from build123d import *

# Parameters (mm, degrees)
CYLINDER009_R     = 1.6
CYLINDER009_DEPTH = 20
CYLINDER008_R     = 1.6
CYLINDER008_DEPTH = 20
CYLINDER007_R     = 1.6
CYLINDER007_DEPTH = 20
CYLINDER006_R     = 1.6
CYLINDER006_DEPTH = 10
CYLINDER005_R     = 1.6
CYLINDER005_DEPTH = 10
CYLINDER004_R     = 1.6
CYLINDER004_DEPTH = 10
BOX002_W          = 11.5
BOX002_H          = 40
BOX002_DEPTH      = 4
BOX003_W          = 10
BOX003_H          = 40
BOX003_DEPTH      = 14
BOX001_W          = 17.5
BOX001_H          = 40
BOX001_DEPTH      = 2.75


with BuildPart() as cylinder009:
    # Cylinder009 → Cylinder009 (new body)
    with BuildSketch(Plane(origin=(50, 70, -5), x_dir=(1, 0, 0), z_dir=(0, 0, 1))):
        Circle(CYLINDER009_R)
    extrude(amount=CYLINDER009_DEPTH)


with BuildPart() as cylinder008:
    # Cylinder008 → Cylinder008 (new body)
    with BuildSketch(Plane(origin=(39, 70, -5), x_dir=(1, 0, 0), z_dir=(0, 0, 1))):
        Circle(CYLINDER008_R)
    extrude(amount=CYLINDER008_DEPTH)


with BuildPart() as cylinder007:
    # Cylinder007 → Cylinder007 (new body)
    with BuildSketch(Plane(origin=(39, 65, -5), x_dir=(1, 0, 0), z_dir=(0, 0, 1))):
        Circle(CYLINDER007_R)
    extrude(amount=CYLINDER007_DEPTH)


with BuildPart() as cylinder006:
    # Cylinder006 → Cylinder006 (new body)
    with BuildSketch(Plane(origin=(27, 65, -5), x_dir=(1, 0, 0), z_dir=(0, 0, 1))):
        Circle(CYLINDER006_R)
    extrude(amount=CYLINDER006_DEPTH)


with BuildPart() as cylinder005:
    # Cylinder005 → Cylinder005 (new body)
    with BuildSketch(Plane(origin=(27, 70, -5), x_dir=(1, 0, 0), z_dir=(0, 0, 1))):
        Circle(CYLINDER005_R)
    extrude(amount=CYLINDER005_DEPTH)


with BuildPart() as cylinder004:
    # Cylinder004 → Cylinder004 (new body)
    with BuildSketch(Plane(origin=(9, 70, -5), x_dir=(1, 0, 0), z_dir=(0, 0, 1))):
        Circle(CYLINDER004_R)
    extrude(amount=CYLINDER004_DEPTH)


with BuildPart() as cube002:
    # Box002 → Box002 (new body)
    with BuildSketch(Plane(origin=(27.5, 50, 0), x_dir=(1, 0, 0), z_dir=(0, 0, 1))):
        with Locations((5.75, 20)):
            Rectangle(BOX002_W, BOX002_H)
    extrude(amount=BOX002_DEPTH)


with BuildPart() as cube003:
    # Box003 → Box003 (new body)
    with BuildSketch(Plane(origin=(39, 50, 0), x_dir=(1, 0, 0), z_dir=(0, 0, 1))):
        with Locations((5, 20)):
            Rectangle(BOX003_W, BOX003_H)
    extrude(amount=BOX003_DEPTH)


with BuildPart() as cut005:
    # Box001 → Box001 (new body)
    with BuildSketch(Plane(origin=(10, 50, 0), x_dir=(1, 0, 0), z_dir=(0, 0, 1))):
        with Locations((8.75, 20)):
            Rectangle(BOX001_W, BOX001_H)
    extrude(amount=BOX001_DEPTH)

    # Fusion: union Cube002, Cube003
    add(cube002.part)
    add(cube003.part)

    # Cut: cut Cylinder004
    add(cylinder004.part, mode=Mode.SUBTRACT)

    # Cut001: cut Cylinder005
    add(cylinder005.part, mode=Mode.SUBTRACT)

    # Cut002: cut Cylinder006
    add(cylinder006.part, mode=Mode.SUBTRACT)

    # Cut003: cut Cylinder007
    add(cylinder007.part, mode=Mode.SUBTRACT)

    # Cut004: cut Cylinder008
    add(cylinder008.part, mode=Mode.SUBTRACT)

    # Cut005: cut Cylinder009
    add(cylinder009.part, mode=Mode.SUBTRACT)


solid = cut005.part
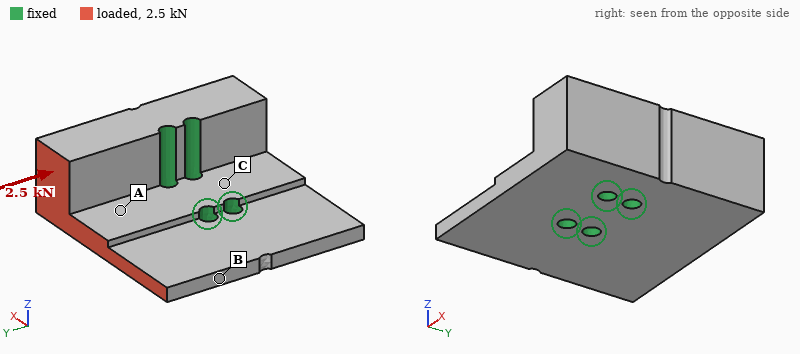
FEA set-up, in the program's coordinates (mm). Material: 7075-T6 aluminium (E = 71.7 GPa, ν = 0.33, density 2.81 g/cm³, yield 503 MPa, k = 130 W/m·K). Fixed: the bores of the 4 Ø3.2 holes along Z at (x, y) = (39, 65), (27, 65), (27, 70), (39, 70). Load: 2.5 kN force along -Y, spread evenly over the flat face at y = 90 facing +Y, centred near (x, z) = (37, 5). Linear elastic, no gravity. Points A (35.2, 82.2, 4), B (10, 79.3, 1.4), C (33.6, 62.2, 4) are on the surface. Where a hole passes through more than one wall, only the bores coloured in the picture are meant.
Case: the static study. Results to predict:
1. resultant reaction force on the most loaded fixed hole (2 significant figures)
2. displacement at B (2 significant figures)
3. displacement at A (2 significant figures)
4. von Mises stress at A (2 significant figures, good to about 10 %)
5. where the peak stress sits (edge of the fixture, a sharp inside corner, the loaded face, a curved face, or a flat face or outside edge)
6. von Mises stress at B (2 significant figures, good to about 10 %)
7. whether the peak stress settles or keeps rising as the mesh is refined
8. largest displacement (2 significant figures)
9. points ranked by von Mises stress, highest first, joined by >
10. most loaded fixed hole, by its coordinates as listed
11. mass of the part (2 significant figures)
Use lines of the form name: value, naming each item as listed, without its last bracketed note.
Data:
resultant reaction force on the most loaded fixed hole: 1.3 kN
displacement at B: 4.4 µm
displacement at A: 2.3 µm
von Mises stress at A: 13 MPa
where the peak stress sits: edge of the fixture
von Mises stress at B: 8.3 MPa
whether the peak stress settles or keeps rising as the mesh is refined: keeps rising
largest displacement: 6.6 µm
points ranked by von Mises stress, highest first, joined by >: A > B > C
most loaded fixed hole, by its coordinates as listed: (39, 70)
mass of the part: 26 g
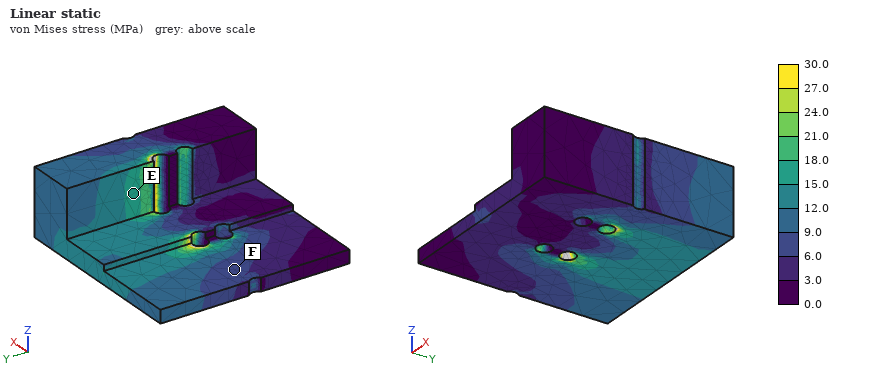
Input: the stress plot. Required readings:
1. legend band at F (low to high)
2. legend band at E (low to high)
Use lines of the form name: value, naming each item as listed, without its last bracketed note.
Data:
legend band at F: 6.0 to 9.0 MPa
legend band at E: 15.0 to 18.0 MPa
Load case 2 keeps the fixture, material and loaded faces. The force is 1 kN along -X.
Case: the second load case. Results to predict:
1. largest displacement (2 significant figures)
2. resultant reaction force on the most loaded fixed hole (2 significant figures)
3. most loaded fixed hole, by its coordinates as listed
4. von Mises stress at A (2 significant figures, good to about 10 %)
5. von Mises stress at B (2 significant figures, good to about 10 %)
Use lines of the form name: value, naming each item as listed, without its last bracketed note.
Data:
largest displacement: 19 µm
resultant reaction force on the most loaded fixed hole: 1.3 kN
most loaded fixed hole, by its coordinates as listed: (39, 70)
von Mises stress at A: 22 MPa
von Mises stress at B: 7.6 MPa
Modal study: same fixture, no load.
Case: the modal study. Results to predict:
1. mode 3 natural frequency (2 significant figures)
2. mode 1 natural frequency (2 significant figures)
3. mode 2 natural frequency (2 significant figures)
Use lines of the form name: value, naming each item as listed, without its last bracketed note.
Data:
mode 3 natural frequency: 14 kHz
mode 1 natural frequency: 6500 Hz
mode 2 natural frequency: 7900 Hz
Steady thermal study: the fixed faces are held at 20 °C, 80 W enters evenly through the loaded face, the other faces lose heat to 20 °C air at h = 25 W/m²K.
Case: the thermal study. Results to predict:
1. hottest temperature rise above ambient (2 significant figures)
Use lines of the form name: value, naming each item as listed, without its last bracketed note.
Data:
hottest temperature rise above ambient: 60 K
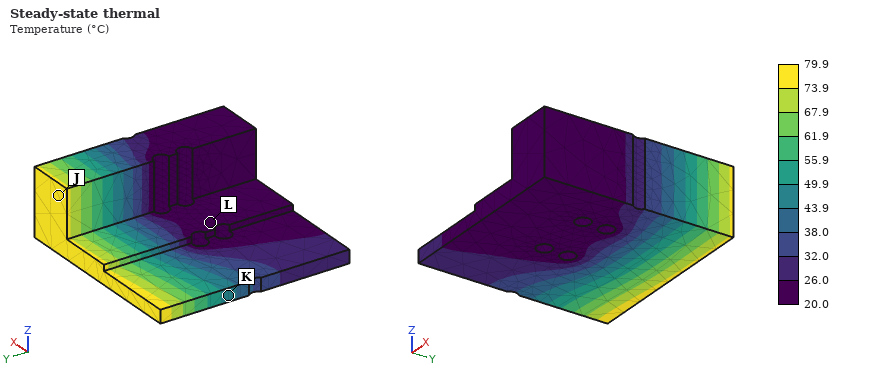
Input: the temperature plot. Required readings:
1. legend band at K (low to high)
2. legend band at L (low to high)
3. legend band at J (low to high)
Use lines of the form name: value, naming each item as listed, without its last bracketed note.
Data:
legend band at K: 43.9 to 49.9 °C
legend band at L: 20.0 to 26.0 °C
legend band at J: 73.9 to 79.9 °C
